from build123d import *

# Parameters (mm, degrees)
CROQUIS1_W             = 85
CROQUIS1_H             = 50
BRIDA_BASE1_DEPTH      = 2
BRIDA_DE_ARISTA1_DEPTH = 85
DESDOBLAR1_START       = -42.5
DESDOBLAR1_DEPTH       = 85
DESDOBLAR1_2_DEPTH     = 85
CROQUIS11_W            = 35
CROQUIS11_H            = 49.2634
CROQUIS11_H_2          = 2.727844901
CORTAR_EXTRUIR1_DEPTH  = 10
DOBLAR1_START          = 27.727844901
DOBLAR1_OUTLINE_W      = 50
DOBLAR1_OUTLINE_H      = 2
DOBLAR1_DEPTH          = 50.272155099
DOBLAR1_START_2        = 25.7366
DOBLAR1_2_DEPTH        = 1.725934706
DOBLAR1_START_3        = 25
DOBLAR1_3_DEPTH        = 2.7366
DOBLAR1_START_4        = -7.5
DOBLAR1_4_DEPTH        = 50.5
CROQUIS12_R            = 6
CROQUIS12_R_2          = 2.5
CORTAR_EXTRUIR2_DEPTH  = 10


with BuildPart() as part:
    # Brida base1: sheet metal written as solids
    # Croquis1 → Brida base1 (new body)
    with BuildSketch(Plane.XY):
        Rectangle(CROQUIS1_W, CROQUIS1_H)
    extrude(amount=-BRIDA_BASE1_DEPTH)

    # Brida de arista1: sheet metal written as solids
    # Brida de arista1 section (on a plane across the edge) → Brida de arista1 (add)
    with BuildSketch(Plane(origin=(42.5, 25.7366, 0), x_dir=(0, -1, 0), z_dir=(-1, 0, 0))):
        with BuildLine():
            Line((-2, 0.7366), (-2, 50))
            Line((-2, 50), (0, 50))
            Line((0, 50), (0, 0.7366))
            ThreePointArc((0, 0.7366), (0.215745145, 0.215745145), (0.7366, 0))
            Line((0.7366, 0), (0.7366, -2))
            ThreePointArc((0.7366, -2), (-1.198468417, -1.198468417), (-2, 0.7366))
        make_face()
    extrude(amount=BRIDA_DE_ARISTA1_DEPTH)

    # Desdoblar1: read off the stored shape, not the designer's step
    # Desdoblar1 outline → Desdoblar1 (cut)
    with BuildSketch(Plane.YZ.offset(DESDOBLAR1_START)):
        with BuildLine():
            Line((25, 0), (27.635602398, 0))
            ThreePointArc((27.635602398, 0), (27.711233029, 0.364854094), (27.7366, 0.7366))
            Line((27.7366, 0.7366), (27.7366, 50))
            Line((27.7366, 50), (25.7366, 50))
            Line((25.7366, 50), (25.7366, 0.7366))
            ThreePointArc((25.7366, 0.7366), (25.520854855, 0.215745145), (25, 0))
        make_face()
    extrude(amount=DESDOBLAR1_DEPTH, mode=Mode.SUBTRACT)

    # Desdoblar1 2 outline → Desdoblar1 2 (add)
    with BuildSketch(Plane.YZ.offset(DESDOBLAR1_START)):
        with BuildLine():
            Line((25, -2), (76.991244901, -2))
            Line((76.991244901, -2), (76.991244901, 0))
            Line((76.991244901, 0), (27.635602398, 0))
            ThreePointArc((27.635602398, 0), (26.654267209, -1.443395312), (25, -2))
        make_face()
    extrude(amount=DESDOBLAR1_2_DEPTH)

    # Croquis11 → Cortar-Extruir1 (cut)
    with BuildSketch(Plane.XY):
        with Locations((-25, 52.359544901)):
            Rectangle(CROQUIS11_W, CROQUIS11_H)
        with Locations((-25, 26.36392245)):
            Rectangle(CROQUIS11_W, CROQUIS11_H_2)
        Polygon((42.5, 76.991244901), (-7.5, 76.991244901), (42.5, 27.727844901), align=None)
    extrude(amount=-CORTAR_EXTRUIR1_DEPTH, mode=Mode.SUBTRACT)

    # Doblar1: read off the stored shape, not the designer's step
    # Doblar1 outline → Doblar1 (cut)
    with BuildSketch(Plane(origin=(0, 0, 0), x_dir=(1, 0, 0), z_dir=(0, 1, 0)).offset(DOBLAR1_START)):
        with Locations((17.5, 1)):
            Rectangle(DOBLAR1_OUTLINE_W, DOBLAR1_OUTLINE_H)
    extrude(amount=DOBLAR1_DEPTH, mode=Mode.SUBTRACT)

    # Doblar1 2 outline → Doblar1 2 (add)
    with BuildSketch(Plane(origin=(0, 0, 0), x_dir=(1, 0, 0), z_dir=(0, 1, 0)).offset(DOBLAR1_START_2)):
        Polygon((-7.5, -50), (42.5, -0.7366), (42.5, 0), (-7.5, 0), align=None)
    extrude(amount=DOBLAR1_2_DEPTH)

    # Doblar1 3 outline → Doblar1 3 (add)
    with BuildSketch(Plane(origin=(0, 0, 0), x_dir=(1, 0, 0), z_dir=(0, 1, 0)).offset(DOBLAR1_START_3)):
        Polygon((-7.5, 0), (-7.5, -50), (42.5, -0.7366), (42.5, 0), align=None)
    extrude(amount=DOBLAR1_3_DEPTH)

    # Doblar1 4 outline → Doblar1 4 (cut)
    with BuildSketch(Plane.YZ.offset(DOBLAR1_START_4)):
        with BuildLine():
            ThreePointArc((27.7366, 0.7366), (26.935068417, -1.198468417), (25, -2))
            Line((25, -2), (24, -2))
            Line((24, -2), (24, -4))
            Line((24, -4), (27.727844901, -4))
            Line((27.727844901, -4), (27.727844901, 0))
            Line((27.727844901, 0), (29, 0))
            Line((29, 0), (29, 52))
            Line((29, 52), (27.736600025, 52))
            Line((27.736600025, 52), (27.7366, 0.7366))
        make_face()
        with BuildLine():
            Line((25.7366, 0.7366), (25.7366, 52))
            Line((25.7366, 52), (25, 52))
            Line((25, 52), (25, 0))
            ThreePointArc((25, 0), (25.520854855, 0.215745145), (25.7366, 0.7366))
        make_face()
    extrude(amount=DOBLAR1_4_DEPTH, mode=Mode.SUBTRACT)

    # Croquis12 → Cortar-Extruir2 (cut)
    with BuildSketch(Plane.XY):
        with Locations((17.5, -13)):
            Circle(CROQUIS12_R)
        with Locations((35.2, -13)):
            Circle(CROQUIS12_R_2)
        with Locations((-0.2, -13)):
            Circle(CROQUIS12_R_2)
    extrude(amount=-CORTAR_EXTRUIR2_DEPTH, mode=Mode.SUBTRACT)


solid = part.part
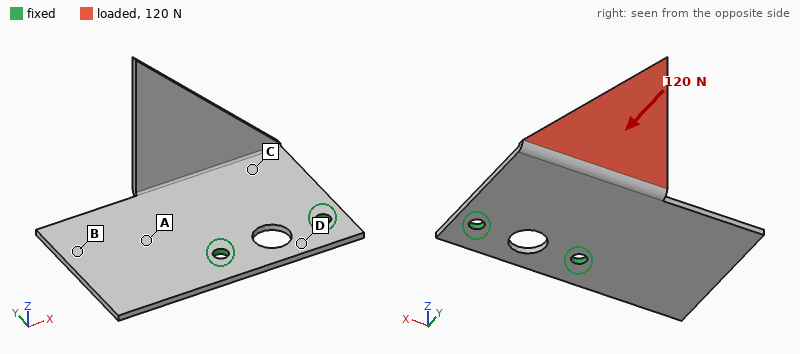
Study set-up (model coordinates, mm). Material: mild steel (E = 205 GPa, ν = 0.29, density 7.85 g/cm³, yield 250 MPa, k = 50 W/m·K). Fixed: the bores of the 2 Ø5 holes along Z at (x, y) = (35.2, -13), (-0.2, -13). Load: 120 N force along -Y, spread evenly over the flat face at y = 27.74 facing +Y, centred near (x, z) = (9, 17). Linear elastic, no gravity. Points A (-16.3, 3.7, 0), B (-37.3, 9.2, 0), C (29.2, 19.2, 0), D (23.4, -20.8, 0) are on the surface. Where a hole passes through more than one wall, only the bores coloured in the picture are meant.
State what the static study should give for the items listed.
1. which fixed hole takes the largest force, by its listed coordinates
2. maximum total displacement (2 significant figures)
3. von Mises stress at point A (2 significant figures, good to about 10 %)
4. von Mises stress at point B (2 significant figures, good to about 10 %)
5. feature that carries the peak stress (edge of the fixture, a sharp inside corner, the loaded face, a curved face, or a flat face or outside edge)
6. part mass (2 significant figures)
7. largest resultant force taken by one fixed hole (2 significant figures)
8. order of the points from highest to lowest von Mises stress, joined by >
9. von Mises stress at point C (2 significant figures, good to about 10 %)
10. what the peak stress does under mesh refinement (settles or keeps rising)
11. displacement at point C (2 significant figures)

(-0.2, -13)
0.77 mm
32 MPa
15 MPa
a sharp inside corner
86 g
88 N
C > A > B > D
45 MPa
keeps rising
0.13 mm
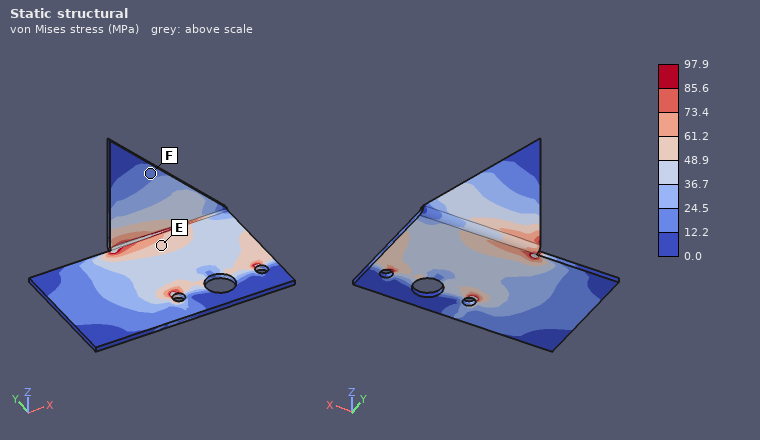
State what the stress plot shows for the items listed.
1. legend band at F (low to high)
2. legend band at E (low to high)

12.2 to 24.5 MPa
48.9 to 61.2 MPa
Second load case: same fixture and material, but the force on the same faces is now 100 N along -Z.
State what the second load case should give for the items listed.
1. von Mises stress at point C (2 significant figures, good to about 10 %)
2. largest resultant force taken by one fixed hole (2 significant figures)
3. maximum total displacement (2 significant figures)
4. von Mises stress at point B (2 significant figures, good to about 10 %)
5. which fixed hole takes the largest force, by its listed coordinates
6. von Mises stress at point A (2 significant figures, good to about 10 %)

19 MPa
69 N
0.55 mm
17 MPa
(-0.2, -13)
38 MPa
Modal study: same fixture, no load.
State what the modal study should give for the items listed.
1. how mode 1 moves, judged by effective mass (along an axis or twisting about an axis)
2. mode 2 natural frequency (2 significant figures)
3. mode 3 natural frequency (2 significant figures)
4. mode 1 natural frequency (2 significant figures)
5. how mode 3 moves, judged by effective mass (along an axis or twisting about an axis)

along Z
740 Hz
1100 Hz
470 Hz
along Z
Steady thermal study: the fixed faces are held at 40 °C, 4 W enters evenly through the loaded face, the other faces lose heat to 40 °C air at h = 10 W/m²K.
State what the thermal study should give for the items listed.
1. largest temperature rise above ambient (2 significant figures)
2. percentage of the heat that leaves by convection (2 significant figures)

43 K
31 %
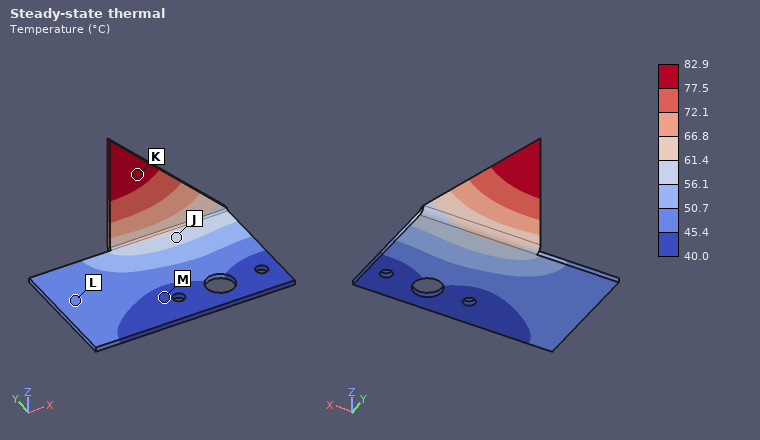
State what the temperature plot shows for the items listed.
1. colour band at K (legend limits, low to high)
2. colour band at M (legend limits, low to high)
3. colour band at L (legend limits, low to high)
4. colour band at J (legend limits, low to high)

77.5 to 82.9 °C
40.0 to 45.4 °C
45.4 to 50.7 °C
56.1 to 61.4 °C
